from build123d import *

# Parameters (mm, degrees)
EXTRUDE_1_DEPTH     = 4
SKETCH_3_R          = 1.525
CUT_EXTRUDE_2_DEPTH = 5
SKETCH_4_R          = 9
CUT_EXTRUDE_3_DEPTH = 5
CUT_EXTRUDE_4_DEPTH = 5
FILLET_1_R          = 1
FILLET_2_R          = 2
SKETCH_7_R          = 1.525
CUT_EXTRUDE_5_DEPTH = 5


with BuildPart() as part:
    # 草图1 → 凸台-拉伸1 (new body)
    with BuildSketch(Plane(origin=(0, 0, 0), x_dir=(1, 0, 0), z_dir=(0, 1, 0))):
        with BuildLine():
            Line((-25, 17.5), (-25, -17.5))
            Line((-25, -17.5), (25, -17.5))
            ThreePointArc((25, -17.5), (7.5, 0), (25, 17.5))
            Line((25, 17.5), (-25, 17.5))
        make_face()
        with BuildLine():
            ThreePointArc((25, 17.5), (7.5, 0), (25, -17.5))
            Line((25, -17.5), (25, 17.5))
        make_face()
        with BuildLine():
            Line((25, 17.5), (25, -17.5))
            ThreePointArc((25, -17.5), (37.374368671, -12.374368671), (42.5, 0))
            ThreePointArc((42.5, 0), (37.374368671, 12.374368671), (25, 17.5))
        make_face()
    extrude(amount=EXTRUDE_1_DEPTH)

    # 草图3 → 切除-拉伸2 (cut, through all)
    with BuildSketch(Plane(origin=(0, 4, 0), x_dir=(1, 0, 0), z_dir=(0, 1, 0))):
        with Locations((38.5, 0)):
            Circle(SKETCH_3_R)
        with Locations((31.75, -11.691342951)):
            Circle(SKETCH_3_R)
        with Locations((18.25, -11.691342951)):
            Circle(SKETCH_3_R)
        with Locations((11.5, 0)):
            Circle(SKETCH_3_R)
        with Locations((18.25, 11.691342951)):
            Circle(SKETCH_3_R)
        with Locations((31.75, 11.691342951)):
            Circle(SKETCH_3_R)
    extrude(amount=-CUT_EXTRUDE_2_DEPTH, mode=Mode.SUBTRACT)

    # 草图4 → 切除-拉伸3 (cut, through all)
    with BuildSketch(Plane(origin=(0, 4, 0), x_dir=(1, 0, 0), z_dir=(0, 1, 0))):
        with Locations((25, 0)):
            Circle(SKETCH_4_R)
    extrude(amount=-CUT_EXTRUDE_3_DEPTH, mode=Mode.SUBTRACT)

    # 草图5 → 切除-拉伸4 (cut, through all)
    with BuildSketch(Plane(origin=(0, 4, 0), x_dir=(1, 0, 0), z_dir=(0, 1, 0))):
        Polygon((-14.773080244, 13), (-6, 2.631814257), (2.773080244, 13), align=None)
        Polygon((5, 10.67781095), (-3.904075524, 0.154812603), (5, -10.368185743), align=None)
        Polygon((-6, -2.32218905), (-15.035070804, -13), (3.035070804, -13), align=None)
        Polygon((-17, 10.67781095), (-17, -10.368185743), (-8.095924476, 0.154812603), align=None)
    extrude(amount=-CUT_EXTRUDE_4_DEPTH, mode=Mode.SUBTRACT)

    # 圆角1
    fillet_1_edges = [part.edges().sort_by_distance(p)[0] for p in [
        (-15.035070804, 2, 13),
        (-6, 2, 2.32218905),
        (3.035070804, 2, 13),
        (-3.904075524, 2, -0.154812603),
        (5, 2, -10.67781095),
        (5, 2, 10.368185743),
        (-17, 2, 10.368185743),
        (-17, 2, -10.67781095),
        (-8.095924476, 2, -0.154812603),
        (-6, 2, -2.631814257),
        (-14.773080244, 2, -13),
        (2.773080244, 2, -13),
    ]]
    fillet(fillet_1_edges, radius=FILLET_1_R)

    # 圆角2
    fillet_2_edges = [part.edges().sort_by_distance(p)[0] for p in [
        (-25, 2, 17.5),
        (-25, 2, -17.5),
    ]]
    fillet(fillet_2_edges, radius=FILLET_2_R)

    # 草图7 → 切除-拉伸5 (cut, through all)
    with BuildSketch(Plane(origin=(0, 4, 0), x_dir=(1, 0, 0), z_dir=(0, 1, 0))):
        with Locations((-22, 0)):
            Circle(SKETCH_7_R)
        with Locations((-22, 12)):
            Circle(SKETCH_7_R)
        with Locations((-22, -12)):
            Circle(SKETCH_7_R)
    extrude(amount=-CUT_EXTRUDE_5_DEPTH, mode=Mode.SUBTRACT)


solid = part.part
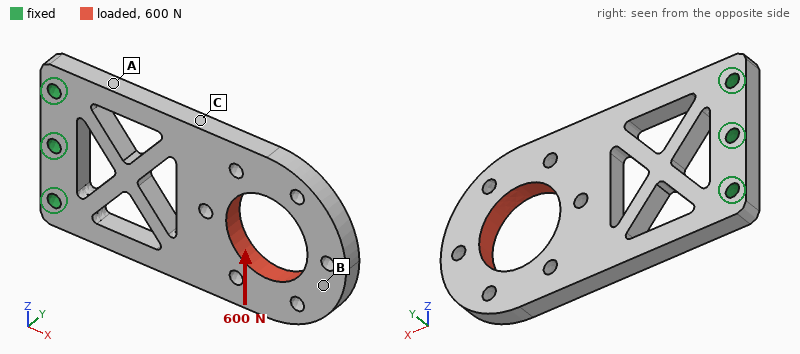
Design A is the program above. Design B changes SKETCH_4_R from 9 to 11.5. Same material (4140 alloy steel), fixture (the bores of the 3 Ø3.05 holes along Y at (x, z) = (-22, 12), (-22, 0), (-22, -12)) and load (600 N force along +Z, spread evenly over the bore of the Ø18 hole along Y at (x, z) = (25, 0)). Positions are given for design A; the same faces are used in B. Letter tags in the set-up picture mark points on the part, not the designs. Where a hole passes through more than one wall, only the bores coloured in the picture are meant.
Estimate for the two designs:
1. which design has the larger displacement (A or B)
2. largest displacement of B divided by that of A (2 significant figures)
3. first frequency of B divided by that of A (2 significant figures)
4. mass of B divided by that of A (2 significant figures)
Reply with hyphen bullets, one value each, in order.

- B
- 1.3
- 1.1
- 0.90
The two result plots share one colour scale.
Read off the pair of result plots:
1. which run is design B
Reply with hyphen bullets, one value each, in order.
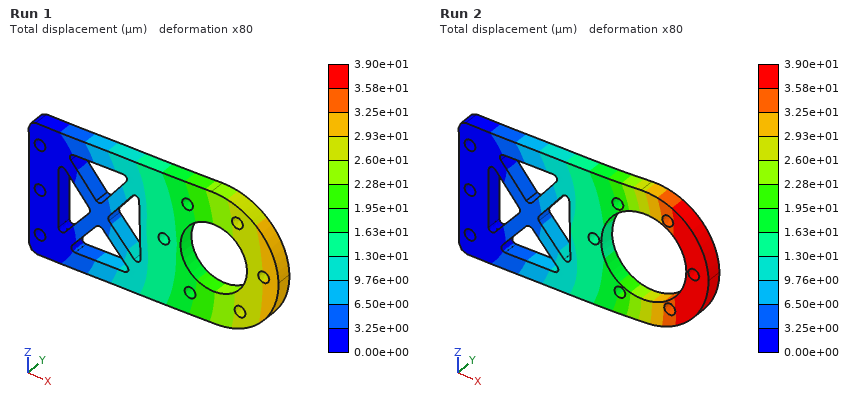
- Run 2
